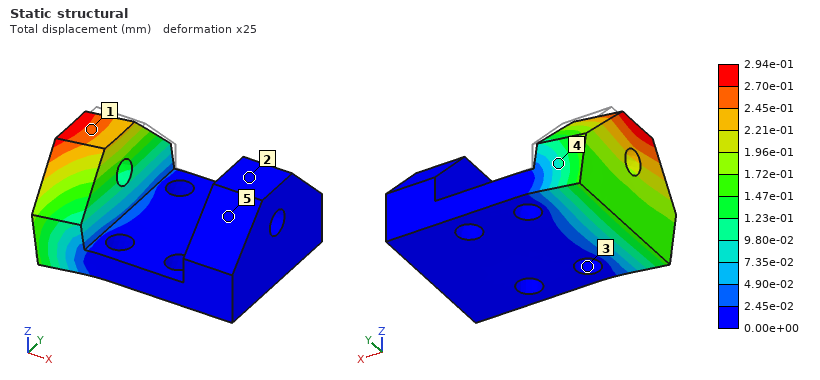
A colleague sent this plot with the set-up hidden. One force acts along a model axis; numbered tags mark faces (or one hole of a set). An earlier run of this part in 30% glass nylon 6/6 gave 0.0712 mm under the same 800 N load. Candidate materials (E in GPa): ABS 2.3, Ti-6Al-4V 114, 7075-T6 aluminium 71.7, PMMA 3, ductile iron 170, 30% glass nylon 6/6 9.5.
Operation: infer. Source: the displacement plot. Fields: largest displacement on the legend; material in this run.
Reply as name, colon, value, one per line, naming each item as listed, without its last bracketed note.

largest displacement on the legend: 2.94e-01 mm
material in this run: ABS
